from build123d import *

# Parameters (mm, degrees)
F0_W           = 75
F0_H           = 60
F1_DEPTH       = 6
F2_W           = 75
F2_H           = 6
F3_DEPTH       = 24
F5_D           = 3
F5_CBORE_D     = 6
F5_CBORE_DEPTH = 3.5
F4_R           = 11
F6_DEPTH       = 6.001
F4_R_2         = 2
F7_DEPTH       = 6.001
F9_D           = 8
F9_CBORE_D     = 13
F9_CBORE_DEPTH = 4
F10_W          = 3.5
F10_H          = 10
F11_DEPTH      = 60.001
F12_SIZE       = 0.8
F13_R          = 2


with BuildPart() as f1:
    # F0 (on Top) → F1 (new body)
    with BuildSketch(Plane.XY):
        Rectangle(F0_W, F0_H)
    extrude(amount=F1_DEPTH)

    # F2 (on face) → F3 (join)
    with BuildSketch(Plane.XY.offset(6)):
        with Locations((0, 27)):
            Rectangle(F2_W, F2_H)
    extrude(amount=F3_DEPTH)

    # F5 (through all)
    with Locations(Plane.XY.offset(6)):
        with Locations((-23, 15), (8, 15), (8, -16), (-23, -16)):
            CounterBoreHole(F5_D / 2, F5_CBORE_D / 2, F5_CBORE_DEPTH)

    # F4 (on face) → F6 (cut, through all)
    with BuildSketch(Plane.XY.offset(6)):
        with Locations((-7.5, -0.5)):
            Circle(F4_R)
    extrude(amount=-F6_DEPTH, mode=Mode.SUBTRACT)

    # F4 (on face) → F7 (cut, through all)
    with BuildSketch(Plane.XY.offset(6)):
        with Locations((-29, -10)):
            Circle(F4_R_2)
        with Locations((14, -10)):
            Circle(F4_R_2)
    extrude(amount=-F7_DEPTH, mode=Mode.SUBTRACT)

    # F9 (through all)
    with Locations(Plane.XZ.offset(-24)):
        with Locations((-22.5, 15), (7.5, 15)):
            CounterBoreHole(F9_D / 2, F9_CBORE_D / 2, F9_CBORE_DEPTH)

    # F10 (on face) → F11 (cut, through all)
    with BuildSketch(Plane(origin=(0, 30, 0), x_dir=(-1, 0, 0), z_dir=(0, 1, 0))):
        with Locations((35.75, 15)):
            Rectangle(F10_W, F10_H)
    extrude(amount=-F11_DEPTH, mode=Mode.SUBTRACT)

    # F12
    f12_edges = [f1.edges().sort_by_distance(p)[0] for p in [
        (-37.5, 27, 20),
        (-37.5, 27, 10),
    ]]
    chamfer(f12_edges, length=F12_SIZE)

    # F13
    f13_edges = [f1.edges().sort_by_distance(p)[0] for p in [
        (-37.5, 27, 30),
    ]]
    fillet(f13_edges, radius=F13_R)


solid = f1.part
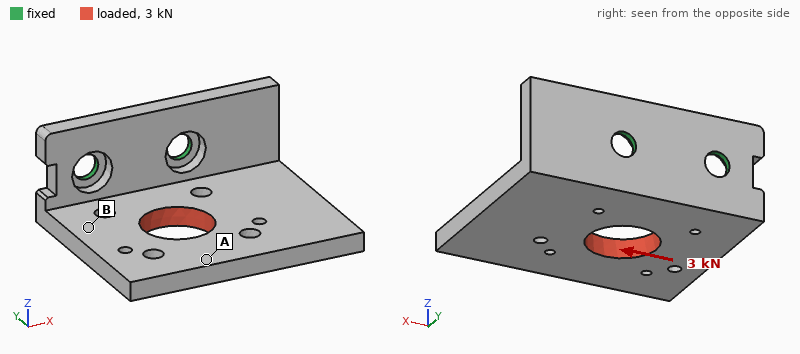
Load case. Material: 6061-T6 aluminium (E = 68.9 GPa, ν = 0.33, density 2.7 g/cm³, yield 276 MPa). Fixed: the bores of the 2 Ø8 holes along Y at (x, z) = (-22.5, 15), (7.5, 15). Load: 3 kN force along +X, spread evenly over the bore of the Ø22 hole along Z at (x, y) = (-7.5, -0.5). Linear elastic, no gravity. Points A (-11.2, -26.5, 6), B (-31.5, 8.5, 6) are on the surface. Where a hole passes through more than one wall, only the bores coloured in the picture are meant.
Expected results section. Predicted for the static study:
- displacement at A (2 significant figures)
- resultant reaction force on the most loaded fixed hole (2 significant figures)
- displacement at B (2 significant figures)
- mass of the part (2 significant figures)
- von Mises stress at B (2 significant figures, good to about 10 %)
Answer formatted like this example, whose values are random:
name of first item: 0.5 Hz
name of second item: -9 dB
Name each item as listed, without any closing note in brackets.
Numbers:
displacement at A: 0.21 mm
resultant reaction force on the most loaded fixed hole: 3.4 kN
displacement at B: 0.12 mm
mass of the part: 90 g
von Mises stress at B: 40 MPa
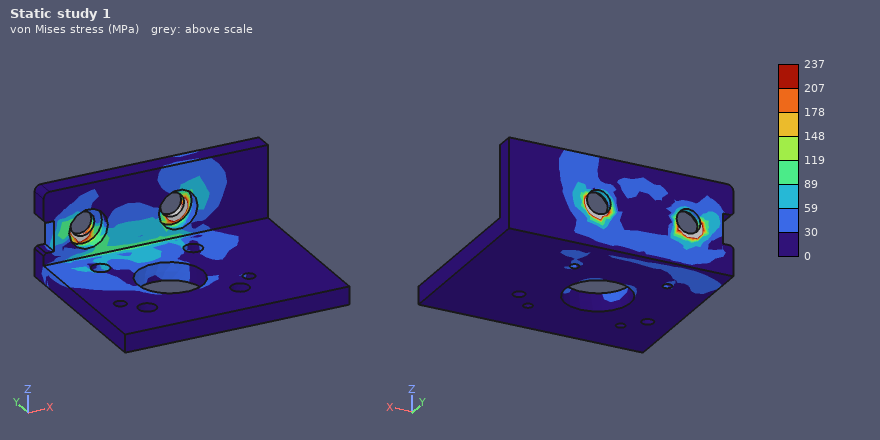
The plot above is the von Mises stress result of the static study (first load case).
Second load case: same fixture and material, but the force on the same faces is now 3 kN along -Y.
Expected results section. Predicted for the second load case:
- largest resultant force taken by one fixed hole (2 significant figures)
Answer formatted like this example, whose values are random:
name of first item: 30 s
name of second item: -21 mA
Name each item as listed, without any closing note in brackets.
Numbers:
largest resultant force taken by one fixed hole: 1.5 kN
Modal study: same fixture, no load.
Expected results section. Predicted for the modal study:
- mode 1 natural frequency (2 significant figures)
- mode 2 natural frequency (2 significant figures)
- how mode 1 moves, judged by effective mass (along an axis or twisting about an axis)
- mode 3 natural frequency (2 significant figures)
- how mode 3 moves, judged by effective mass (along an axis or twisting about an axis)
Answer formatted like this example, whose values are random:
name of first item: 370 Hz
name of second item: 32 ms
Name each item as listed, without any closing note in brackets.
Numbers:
mode 1 natural frequency: 840 Hz
mode 2 natural frequency: 2000 Hz
how mode 1 moves, judged by effective mass: along Z
mode 3 natural frequency: 2800 Hz
how mode 3 moves, judged by effective mass: along X
